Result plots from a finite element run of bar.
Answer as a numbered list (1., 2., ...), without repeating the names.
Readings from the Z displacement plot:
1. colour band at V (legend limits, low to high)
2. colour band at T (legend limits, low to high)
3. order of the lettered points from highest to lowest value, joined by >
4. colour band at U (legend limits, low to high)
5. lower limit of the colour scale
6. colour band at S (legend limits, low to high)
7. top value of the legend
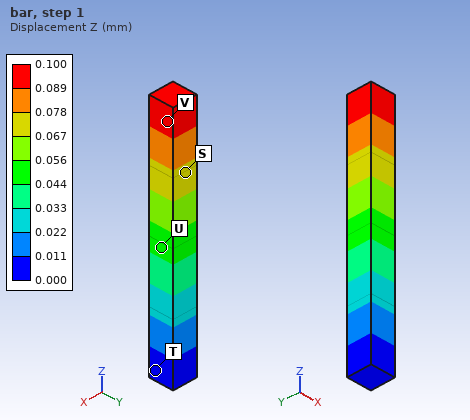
1. 0.089 to 0.100 mm
2. 0.000 to 0.011 mm
3. V > S > U > T
4. 0.044 to 0.056 mm
5. 0.000 mm
6. 0.067 to 0.078 mm
7. 0.100 mm
